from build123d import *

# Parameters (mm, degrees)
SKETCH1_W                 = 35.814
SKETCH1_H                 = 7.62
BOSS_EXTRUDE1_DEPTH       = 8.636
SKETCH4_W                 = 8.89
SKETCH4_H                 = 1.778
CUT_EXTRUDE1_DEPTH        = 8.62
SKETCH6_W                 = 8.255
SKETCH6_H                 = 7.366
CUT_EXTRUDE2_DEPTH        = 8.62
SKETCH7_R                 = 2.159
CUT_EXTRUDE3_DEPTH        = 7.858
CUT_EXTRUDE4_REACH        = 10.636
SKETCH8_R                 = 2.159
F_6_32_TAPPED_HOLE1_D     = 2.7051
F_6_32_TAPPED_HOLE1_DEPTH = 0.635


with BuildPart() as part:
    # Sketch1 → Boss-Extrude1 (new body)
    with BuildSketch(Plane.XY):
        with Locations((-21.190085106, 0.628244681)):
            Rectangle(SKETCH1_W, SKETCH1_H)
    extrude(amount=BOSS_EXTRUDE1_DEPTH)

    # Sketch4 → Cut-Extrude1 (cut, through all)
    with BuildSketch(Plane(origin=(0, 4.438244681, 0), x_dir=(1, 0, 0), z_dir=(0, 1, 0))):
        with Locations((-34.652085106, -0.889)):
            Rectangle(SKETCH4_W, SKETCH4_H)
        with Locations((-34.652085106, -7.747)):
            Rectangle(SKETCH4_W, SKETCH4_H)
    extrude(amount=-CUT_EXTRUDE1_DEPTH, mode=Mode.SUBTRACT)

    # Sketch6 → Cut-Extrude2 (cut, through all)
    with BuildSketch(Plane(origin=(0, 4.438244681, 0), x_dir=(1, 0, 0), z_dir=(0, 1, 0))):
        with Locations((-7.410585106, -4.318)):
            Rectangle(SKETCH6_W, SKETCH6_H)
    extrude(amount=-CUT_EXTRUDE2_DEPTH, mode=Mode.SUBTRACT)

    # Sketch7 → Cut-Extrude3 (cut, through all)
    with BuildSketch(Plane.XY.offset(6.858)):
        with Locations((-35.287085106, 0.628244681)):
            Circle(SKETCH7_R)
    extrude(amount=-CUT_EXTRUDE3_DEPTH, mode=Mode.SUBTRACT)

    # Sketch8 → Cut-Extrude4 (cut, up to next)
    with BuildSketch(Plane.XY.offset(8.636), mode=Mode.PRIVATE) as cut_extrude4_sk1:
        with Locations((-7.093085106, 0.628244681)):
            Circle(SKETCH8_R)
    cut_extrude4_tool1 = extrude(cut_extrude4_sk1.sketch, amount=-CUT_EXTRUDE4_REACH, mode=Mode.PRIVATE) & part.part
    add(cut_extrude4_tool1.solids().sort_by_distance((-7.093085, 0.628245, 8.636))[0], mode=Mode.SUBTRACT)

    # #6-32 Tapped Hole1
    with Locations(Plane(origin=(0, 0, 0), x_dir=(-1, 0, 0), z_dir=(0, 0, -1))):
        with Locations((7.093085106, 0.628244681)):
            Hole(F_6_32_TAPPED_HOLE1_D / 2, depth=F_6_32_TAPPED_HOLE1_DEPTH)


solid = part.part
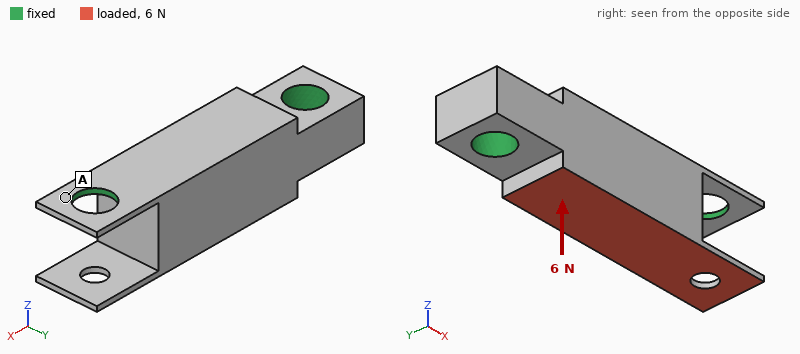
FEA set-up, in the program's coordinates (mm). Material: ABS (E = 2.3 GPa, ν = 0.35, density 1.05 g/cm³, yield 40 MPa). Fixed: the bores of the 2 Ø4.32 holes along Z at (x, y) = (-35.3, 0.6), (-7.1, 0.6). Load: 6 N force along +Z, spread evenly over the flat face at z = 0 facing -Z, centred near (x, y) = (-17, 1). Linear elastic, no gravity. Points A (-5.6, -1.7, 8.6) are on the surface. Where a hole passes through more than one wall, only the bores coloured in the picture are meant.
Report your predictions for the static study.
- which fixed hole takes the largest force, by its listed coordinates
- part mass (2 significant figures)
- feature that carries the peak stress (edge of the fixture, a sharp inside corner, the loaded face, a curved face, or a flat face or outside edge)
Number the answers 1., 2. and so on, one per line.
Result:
1. (-35.3, 0.6)
2. 1.6 g
3. the loaded face
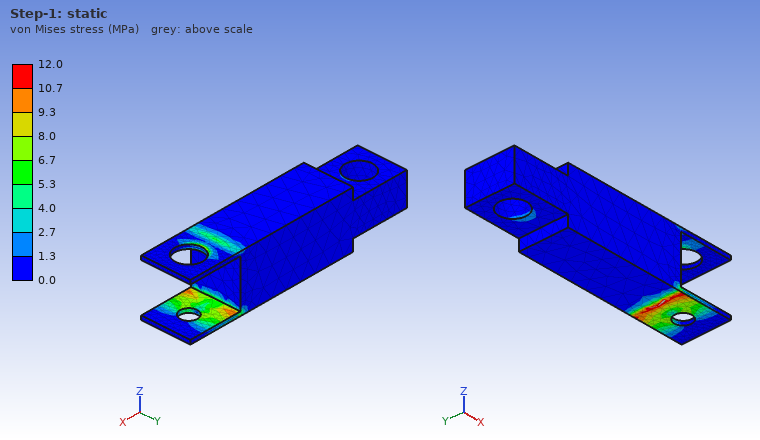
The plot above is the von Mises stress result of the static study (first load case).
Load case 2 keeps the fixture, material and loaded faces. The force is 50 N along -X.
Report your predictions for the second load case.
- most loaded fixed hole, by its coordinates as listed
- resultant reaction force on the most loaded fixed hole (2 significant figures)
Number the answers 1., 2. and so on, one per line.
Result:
1. (-35.3, 0.6)
2. 54 N
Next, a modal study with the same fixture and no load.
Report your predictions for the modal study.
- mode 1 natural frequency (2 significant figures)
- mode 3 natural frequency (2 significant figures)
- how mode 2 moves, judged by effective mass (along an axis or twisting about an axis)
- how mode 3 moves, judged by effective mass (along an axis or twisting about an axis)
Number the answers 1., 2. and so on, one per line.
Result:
1. 2100 Hz
2. 4600 Hz
3. along Z
4. along Y
